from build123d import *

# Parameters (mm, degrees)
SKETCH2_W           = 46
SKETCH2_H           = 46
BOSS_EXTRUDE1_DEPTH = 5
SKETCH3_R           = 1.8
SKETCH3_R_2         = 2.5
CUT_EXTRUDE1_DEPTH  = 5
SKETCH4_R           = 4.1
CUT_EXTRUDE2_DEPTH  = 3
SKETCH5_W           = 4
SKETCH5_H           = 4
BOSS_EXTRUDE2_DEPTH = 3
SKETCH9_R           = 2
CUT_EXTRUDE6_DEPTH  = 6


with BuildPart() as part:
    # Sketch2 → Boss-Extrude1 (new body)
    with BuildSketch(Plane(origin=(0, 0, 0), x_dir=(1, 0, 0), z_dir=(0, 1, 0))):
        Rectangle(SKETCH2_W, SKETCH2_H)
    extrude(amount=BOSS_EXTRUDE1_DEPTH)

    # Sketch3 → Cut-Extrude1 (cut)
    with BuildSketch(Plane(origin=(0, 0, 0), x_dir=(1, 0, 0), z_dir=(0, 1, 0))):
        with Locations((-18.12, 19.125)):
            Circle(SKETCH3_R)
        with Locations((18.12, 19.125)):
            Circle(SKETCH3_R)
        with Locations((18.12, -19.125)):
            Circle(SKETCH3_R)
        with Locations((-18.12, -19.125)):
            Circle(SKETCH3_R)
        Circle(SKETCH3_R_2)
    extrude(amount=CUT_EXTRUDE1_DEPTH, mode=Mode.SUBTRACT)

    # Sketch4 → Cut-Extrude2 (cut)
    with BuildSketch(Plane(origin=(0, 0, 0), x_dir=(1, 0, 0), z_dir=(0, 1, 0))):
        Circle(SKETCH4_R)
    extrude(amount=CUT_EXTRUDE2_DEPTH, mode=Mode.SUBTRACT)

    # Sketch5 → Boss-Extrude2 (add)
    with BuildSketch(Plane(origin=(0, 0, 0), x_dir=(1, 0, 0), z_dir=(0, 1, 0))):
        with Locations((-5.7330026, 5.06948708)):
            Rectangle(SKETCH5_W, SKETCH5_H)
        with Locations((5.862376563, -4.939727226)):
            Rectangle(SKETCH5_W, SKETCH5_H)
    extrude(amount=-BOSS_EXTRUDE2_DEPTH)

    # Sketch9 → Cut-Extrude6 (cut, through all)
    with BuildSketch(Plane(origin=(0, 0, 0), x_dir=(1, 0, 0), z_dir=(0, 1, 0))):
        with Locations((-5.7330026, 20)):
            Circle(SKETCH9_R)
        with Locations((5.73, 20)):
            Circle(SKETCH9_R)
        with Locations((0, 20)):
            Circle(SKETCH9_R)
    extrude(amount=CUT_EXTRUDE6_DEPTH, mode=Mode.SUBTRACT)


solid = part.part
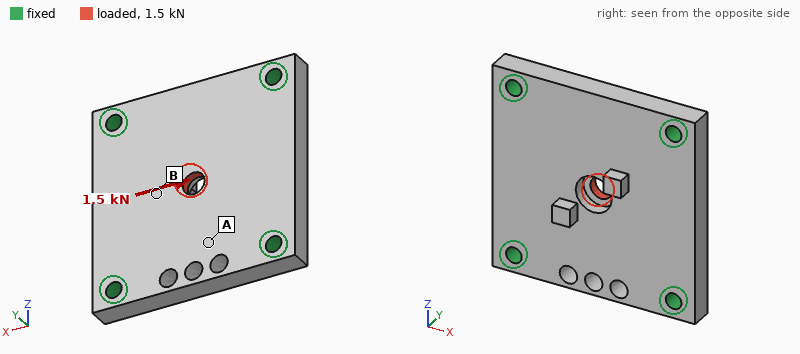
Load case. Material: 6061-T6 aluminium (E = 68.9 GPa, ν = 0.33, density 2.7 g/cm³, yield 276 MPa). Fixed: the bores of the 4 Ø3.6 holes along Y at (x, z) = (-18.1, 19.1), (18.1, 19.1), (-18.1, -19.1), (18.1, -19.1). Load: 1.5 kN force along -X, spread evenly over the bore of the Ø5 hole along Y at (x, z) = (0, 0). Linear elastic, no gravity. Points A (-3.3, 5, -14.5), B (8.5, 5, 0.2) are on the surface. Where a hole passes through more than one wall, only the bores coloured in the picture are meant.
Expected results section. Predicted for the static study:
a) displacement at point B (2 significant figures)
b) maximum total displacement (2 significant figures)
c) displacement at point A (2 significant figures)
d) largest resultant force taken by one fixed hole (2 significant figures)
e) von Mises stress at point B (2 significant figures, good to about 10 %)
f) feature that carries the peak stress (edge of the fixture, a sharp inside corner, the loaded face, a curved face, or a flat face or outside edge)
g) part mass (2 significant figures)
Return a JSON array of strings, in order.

["3.5 µm", "6.3 µm", "1.5 µm", "430 N", "16 MPa", "the loaded face", "27 g"]
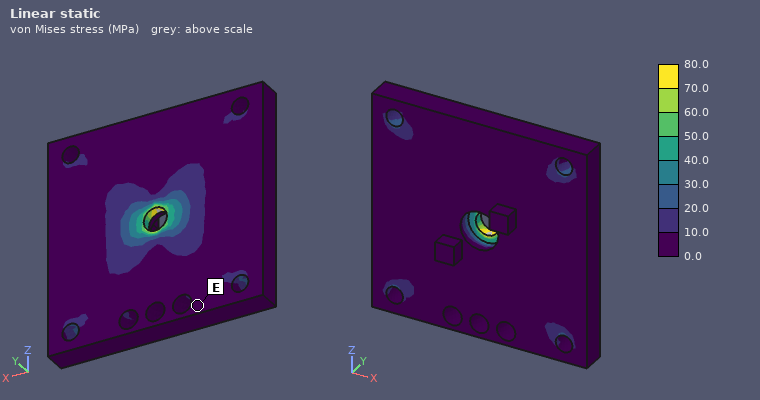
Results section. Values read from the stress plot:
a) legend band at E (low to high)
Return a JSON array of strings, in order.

["0.0 to 10.0 MPa"]
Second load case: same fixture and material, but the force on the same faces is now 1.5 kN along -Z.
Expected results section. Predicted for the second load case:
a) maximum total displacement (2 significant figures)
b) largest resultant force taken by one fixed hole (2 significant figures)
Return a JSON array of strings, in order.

["6.2 µm", "430 N"]
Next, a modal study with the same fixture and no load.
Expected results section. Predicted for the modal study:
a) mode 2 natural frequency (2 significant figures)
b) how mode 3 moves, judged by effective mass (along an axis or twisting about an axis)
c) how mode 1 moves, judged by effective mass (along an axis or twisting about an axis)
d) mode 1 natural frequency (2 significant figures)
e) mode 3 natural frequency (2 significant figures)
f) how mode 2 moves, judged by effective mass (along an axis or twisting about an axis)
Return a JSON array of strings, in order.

["18 kHz", "twisting about X", "along Y", "12 kHz", "20 kHz", "twisting about Z"]
